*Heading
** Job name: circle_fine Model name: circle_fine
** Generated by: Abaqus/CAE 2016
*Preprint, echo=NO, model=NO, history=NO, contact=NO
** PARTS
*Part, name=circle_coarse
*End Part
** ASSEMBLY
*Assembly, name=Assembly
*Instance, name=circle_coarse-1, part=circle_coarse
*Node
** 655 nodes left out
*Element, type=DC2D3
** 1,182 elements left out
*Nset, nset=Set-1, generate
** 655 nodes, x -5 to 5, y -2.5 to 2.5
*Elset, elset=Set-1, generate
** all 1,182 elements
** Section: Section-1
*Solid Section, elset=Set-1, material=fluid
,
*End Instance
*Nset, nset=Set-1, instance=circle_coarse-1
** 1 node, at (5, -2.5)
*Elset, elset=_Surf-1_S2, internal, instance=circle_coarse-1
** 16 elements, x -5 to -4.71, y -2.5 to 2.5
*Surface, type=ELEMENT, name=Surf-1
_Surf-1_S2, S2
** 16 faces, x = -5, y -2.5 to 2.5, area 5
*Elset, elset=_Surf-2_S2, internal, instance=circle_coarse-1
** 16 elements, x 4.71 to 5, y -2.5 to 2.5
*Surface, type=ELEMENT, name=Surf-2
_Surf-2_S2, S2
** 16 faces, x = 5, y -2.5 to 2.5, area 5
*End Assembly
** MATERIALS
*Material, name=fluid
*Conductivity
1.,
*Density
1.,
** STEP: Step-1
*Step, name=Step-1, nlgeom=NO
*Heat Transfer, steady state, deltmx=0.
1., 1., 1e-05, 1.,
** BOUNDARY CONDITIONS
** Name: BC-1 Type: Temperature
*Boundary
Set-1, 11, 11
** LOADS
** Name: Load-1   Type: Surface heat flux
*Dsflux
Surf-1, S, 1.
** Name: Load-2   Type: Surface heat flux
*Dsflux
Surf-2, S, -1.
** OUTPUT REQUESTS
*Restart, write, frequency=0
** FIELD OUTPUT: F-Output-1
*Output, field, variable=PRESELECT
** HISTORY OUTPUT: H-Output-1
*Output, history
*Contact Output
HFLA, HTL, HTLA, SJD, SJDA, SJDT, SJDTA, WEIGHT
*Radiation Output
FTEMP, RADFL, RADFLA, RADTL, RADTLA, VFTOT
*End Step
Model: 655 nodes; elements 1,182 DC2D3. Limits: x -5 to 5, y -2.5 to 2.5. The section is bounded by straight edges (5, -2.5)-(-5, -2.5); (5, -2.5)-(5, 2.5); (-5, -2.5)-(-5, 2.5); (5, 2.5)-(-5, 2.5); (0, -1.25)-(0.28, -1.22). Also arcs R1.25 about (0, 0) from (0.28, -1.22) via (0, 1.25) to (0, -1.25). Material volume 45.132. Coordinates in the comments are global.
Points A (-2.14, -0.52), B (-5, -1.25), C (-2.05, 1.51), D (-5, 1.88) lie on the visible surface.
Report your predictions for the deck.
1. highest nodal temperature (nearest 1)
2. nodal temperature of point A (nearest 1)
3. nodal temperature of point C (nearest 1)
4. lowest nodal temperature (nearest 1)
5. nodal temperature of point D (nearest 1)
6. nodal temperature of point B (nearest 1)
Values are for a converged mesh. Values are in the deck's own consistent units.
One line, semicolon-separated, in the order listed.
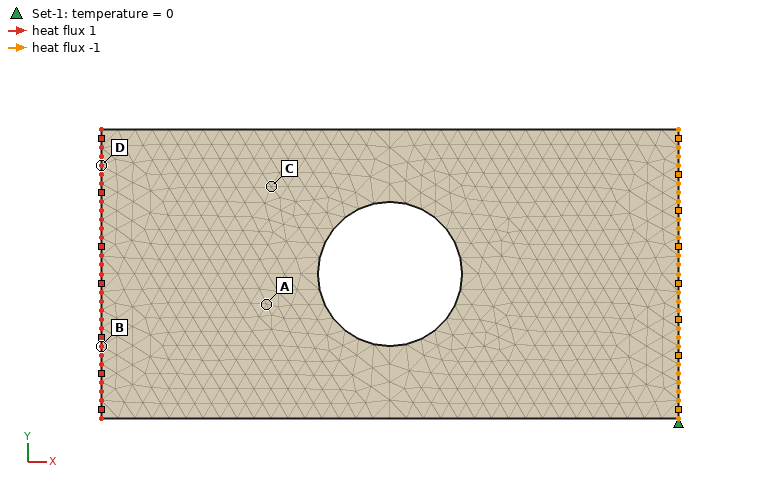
12; 10; 9; 0; 12; 12
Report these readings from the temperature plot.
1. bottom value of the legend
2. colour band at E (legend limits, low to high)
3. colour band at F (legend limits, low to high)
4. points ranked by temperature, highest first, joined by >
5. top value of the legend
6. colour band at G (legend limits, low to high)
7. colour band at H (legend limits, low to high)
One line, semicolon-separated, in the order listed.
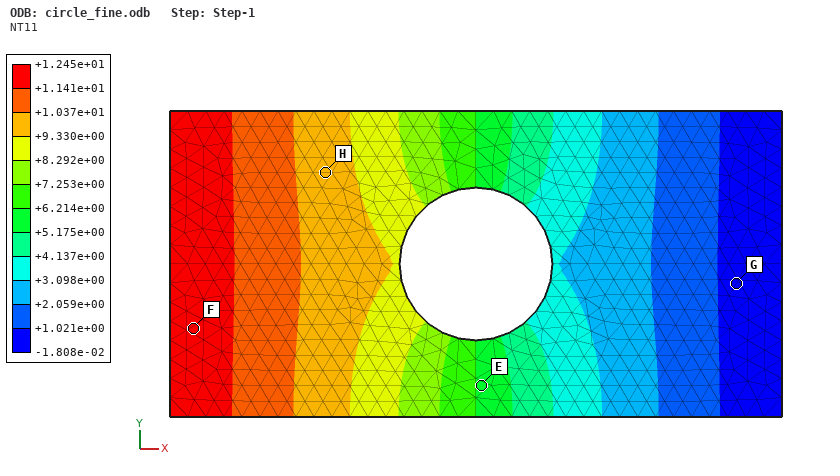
-1.808e-02; +5.175e+00 to +6.214e+00; +1.141e+01 to +1.245e+01; F > H > E > G; +1.245e+01; -1.808e-02 to +1.021e+00; +9.330e+00 to +1.037e+01
